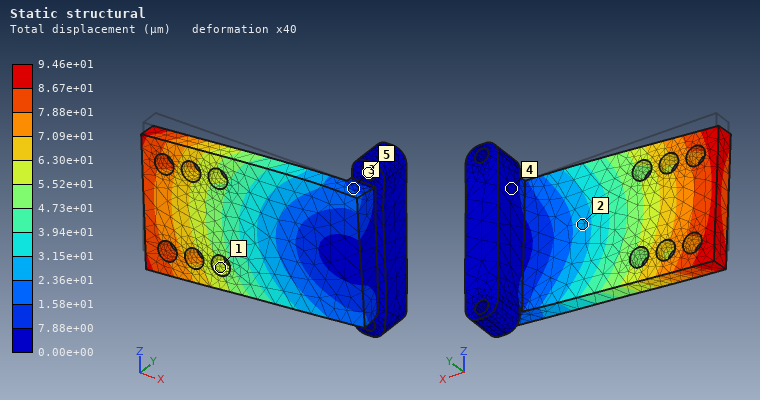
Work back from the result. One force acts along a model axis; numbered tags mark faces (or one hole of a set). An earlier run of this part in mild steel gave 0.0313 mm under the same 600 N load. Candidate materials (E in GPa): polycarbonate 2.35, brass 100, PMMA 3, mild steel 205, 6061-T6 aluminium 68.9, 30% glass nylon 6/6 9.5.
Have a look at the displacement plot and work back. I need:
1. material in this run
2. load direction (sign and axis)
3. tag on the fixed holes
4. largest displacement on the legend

6061-T6 aluminium
-Z
5
9.46e+01 µm
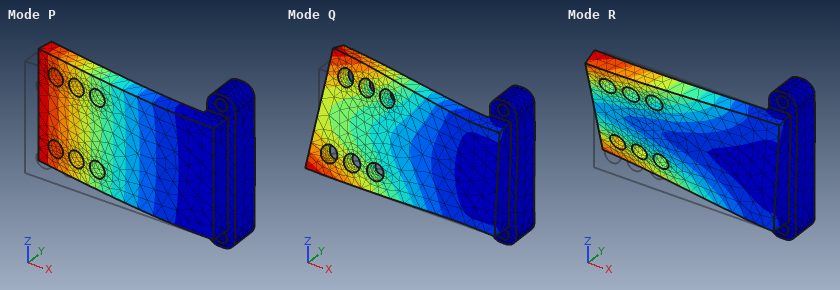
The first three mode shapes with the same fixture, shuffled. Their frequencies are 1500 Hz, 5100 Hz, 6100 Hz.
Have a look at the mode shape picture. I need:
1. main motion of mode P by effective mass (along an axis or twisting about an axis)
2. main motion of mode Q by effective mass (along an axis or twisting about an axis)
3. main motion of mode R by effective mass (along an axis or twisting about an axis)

along Y
along Z
along Z
